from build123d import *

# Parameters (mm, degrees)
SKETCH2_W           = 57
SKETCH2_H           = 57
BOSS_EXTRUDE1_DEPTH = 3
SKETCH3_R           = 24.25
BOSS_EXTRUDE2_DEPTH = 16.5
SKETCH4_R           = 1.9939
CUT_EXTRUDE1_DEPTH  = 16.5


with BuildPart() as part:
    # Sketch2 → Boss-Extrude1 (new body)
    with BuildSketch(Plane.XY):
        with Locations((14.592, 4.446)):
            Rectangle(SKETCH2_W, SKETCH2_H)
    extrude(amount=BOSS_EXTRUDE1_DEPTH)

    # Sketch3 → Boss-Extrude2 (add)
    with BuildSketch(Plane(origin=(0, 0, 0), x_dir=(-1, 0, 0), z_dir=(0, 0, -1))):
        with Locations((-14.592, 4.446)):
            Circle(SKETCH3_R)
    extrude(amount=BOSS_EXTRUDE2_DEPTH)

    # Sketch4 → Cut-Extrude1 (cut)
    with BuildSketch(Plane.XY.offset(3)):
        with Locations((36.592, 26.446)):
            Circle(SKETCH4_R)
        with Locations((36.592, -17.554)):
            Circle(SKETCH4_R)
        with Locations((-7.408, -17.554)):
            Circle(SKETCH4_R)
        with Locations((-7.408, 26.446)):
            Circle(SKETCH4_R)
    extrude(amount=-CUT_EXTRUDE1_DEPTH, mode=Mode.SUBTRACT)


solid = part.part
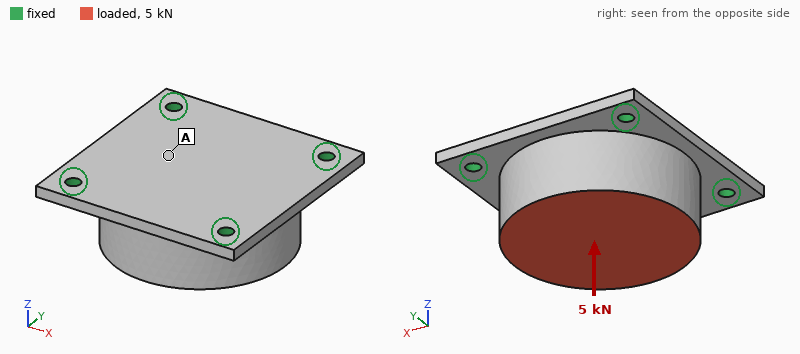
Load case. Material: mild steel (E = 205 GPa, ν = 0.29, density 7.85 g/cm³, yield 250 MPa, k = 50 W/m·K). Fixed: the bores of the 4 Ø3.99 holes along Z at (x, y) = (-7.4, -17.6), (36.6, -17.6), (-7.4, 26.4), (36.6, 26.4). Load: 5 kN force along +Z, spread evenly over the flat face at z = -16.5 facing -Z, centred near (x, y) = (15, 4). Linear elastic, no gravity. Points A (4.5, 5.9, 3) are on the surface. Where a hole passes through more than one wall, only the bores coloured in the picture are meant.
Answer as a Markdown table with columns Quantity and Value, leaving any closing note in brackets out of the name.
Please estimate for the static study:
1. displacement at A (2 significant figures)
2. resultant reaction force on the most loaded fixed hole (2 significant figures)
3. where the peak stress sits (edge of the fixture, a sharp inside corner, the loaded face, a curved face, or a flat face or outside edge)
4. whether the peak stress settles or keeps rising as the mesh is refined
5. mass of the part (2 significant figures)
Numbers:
| Quantity | Value |
|---|---|
| displacement at A | 11 µm |
| resultant reaction force on the most loaded fixed hole | 1.4 kN |
| where the peak stress sits | edge of the fixture |
| whether the peak stress settles or keeps rising as the mesh is refined | keeps rising |
| mass of the part | 310 g |
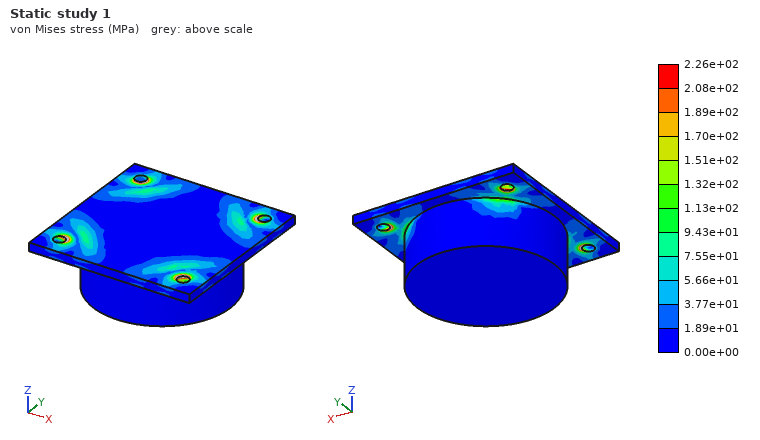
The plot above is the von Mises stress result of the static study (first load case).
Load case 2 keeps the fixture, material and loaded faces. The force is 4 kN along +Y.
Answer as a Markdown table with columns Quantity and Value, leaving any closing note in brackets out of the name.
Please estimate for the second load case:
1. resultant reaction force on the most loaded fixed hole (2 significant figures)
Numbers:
| Quantity | Value |
|---|---|
| resultant reaction force on the most loaded fixed hole | 1.4 kN |
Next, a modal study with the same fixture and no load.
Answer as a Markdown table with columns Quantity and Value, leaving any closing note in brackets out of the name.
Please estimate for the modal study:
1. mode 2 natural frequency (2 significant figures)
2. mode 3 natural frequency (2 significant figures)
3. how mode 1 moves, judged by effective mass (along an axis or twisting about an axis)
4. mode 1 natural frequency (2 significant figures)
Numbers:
| Quantity | Value |
|---|---|
| mode 2 natural frequency | 7500 Hz |
| mode 3 natural frequency | 7600 Hz |
| how mode 1 moves, judged by effective mass | along Z |
| mode 1 natural frequency | 6200 Hz |
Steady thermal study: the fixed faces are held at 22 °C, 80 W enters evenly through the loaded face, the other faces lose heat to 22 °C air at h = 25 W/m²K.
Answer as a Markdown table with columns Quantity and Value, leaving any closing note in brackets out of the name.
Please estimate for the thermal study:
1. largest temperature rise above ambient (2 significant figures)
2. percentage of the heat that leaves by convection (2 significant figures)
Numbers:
| Quantity | Value |
|---|---|
| largest temperature rise above ambient | 79 K |
| percentage of the heat that leaves by convection | 13 % |
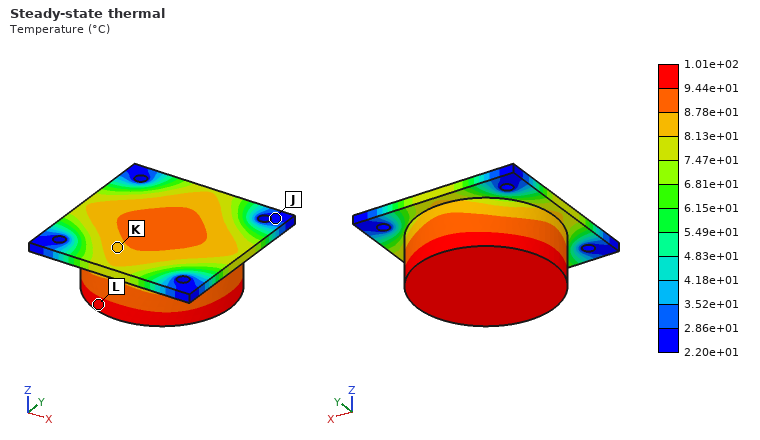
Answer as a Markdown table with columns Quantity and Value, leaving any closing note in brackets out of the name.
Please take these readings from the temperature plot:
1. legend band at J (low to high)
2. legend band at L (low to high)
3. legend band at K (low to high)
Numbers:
| Quantity | Value |
|---|---|
| legend band at J | 2.20e+01 to 2.86e+01 °C |
| legend band at L | 9.44e+01 to 1.01e+02 °C |
| legend band at K | 8.13e+01 to 8.78e+01 °C |
